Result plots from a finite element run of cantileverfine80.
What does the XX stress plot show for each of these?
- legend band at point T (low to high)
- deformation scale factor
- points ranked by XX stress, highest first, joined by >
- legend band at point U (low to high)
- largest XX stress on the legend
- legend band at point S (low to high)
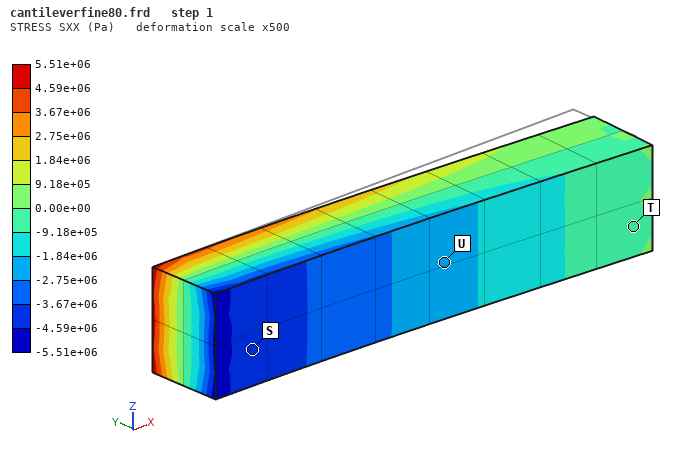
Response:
-9.18e+05 to 0.00e+00 Pa
500
T > U > S
-2.75e+06 to -1.84e+06 Pa
5.51e+06 Pa
-4.59e+06 to -3.67e+06 Pa
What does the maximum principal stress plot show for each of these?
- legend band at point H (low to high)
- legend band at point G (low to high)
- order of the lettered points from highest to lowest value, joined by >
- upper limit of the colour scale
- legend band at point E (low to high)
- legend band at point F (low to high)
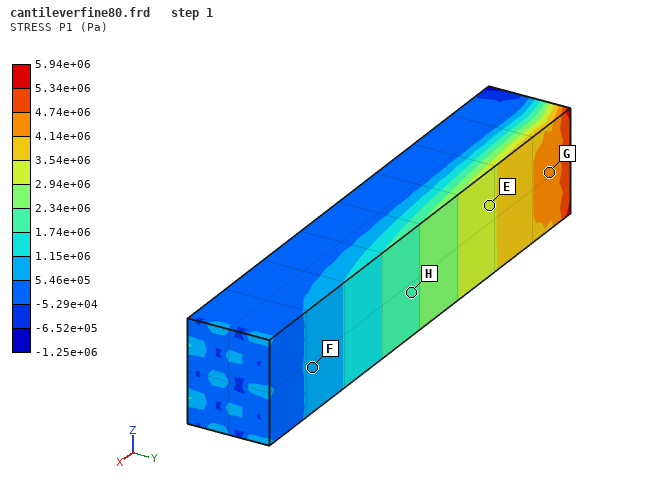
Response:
1.74e+06 to 2.34e+06 Pa
4.14e+06 to 4.74e+06 Pa
G > E > H > F
5.94e+06 Pa
2.94e+06 to 3.54e+06 Pa
5.46e+05 to 1.15e+06 Pa
